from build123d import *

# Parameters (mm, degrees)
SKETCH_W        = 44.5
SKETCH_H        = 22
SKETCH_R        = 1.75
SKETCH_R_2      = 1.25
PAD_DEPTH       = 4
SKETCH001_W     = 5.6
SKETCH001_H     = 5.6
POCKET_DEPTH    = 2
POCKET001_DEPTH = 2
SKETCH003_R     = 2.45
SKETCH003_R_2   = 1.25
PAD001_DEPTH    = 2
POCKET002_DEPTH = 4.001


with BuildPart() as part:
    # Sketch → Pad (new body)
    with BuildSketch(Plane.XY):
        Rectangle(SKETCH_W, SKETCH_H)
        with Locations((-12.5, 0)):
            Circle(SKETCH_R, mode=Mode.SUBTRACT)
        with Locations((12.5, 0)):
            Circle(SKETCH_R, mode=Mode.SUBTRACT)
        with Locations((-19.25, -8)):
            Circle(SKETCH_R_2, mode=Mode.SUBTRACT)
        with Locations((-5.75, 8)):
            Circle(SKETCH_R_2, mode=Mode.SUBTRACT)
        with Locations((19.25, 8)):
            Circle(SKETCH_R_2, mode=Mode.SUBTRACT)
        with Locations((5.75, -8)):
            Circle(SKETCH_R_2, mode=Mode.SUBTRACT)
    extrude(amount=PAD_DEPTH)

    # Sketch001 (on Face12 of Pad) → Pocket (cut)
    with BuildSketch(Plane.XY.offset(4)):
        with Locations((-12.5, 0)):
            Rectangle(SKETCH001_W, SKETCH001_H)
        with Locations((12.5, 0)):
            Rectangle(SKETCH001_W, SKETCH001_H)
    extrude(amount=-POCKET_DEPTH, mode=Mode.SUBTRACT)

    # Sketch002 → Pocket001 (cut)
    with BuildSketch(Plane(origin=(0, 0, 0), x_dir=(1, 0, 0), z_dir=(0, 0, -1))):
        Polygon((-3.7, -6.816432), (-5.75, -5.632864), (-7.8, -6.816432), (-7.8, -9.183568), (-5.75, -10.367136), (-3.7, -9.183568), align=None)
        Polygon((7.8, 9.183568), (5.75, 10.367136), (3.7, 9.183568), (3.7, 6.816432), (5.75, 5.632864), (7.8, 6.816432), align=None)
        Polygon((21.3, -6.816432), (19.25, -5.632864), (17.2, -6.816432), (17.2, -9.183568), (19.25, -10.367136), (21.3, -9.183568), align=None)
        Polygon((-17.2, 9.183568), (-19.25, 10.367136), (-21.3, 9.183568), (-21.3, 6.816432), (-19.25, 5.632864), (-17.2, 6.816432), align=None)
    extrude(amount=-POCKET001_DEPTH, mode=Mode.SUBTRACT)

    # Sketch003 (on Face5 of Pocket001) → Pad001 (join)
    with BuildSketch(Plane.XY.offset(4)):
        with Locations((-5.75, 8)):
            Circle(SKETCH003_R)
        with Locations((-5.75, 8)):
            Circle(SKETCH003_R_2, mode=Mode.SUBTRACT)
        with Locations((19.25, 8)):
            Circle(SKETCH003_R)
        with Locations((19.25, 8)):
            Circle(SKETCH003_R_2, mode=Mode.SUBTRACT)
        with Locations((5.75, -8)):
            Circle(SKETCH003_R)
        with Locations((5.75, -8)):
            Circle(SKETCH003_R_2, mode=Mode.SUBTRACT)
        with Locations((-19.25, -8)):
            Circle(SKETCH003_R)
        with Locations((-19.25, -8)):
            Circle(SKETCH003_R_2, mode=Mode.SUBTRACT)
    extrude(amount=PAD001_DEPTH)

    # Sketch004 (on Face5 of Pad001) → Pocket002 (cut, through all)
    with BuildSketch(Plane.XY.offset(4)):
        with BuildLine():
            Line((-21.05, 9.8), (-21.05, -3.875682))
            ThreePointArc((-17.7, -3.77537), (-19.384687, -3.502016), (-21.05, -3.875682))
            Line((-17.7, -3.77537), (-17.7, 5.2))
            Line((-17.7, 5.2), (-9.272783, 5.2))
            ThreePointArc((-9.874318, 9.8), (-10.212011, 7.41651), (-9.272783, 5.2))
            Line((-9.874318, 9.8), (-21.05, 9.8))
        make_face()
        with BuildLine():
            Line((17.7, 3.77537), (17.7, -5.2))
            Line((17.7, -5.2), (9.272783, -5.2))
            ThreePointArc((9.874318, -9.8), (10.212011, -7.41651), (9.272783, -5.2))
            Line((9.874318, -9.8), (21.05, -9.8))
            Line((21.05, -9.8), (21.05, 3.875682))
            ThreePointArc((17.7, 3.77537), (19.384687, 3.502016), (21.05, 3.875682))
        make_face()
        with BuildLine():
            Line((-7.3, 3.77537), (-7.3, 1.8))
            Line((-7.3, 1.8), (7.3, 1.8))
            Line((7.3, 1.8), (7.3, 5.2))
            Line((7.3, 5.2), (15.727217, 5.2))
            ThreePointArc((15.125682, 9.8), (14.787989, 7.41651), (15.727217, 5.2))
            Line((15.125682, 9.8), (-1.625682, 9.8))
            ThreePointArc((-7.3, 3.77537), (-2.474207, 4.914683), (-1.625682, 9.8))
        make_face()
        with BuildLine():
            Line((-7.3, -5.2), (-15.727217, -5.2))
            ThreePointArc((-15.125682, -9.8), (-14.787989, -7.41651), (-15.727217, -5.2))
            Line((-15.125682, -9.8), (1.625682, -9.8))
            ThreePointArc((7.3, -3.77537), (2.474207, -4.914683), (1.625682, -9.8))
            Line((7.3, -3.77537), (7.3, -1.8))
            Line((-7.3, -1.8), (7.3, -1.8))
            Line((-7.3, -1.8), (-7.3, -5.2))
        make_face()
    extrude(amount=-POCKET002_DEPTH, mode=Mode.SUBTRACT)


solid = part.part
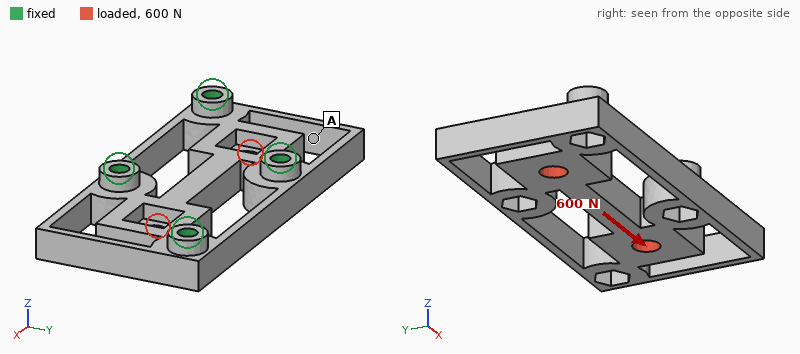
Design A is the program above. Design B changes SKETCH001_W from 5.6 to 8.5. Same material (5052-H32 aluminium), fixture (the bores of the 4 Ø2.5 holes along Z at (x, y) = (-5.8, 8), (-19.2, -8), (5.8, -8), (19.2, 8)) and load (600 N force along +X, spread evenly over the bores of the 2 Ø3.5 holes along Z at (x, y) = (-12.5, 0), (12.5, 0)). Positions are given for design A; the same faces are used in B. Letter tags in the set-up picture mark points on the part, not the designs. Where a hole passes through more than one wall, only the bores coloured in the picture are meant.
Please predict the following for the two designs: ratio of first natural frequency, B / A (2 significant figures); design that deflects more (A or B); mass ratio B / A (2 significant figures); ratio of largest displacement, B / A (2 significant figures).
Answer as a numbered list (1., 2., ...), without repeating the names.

1. 1.00
2. B
3. 0.97
4. 1.1
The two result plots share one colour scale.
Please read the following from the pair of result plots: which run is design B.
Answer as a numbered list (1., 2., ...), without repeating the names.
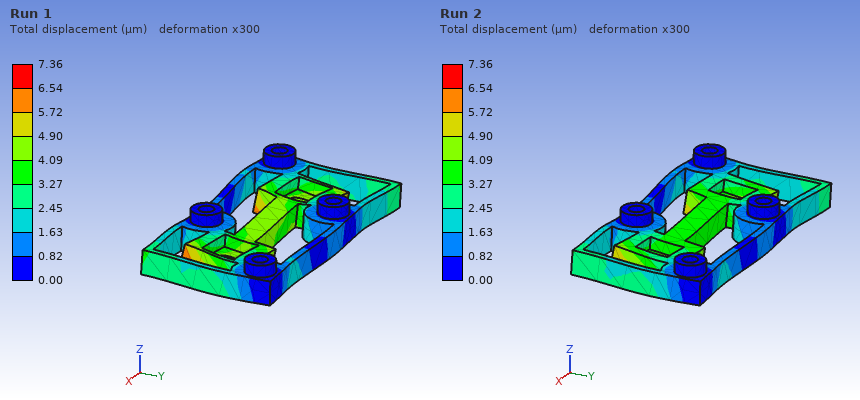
1. Run 1
